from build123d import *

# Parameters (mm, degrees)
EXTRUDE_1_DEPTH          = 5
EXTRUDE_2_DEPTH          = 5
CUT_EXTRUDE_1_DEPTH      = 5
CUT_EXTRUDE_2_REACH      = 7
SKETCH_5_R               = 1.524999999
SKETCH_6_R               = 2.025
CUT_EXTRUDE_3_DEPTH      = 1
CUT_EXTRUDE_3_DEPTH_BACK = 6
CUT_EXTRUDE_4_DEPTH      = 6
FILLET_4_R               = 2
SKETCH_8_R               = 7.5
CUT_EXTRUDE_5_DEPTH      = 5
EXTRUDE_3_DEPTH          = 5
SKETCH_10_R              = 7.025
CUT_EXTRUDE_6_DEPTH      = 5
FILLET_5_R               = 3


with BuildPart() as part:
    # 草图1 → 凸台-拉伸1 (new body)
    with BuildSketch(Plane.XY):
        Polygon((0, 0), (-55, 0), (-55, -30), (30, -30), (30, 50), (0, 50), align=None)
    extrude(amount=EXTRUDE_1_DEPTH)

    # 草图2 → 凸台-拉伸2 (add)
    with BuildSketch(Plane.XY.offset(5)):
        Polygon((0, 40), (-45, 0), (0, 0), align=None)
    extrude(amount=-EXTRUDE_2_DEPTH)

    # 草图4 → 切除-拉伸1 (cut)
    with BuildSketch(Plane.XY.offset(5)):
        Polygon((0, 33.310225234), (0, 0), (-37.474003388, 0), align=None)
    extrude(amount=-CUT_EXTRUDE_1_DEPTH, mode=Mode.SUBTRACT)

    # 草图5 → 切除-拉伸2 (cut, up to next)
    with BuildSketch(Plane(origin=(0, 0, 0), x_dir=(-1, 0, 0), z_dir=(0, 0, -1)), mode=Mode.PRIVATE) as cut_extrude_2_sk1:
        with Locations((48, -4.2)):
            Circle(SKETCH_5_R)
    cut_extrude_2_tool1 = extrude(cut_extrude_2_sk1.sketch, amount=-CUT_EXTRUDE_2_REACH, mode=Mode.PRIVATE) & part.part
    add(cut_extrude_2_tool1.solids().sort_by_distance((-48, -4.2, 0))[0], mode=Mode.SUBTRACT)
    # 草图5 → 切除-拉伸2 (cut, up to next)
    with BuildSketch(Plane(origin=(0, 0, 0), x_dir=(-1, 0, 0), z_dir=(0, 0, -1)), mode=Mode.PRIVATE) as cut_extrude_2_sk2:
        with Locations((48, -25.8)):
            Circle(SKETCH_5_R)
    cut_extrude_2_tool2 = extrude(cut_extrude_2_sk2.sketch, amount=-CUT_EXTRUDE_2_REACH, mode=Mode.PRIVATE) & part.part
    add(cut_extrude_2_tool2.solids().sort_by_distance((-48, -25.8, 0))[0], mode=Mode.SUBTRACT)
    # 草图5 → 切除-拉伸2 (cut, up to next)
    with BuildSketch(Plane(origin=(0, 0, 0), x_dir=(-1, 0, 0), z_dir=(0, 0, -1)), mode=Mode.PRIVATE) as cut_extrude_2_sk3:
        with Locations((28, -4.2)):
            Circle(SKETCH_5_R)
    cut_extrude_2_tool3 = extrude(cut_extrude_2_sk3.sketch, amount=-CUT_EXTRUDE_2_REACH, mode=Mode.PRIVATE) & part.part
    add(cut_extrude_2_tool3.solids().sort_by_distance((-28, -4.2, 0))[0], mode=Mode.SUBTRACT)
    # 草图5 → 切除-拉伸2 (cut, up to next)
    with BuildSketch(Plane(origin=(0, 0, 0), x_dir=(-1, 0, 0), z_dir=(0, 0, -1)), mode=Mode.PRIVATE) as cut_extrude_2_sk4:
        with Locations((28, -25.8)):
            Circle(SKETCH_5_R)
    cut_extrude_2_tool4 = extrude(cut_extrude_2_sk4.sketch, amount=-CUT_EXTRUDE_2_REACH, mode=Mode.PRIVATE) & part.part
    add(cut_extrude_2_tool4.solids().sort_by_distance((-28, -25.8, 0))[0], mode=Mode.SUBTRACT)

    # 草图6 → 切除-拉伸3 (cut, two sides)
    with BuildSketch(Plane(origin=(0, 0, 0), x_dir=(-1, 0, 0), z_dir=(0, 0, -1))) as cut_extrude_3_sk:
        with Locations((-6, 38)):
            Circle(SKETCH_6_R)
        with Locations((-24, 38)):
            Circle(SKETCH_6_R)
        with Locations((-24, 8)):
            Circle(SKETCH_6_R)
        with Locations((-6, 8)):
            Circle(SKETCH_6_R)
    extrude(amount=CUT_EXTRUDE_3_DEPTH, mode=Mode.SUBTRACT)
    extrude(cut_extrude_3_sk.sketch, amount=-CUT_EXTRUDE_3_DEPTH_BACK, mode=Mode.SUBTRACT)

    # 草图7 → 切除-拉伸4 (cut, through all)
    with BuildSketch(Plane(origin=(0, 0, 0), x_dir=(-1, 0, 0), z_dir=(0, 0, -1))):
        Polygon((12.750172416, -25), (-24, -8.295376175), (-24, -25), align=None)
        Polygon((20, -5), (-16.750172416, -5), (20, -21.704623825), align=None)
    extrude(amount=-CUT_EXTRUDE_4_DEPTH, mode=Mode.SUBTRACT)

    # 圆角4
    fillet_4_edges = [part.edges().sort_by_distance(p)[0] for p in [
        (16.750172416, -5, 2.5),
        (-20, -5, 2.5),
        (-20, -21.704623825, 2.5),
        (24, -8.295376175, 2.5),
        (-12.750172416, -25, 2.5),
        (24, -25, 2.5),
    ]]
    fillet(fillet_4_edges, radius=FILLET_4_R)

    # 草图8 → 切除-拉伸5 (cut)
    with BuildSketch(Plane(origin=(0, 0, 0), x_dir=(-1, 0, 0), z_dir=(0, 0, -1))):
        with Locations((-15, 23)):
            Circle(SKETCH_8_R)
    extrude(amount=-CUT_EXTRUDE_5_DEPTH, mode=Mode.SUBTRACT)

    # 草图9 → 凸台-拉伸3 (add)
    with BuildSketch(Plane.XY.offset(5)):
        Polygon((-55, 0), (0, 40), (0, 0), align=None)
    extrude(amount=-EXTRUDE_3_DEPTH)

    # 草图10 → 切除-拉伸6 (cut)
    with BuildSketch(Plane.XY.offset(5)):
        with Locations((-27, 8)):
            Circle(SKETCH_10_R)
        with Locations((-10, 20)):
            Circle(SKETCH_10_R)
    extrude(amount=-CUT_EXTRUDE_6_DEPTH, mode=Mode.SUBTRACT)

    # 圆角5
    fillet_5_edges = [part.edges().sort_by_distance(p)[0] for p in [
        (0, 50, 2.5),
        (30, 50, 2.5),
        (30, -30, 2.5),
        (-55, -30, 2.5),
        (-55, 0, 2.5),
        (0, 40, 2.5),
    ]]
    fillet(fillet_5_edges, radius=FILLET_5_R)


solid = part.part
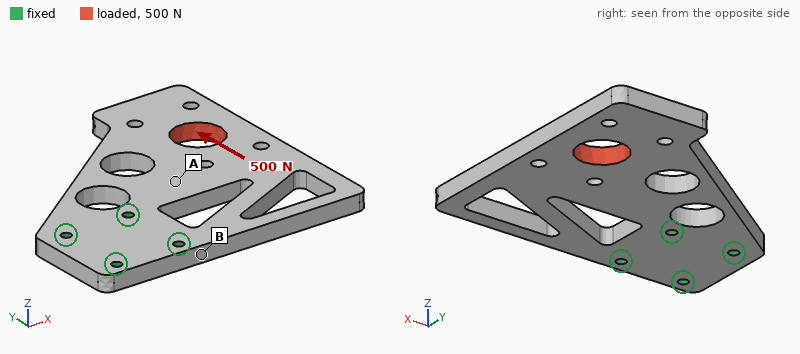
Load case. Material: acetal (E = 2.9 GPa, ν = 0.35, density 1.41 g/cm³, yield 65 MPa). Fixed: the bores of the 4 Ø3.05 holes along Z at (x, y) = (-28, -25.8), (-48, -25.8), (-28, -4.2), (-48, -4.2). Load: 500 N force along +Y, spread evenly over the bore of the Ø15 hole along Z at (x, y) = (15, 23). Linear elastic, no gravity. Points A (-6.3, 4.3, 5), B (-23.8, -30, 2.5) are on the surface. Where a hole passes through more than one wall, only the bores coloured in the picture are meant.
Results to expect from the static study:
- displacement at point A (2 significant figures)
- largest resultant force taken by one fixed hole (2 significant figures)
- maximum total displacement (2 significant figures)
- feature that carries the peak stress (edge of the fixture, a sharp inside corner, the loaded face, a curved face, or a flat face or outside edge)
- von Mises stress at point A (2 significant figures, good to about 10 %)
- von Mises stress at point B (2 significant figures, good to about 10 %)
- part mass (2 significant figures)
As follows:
0.46 mm
690 N
1.3 mm
a curved face
6.4 MPa
22 MPa
28 g
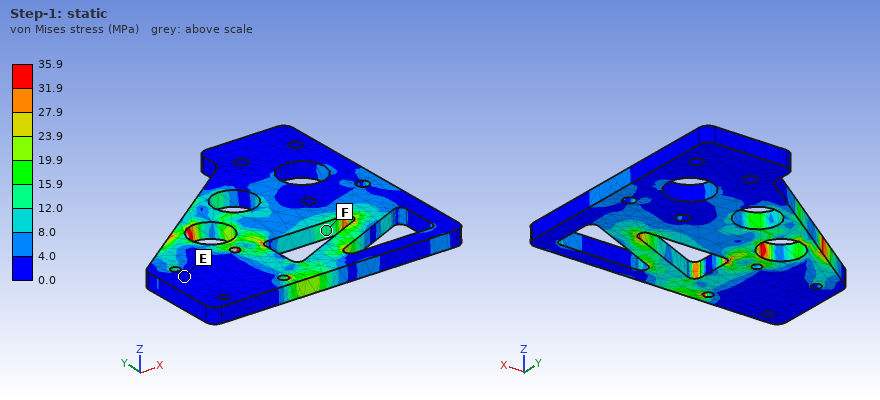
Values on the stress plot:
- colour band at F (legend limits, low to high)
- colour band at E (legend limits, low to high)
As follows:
12.0 to 15.9 MPa
0.0 to 4.0 MPa
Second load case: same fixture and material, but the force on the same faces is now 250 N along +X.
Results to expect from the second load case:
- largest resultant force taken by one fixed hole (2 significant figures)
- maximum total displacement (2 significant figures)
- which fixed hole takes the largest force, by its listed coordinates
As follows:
300 N
0.44 mm
(-28, -4.2)
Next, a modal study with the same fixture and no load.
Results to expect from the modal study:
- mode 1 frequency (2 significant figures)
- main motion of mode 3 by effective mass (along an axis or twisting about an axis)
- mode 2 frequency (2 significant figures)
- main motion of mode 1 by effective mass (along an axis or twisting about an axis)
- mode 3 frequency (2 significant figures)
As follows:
170 Hz
along Y
400 Hz
along Z
900 Hz
